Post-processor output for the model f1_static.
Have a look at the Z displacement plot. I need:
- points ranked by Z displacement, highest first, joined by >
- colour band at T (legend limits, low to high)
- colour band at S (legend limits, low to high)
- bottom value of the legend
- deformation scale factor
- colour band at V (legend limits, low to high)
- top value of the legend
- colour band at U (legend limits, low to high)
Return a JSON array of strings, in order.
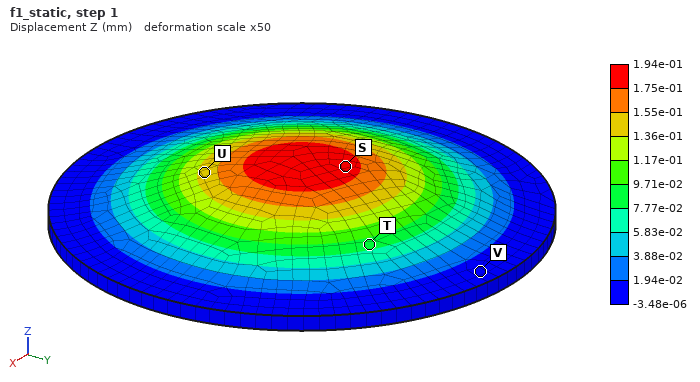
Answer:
["S > U > T > V", "7.77e-02 to 9.71e-02 mm", "1.75e-01 to 1.94e-01 mm", "-3.48e-06 mm", "50", "-3.48e-06 to 1.94e-02 mm", "1.94e-01 mm", "1.36e-01 to 1.55e-01 mm"]
